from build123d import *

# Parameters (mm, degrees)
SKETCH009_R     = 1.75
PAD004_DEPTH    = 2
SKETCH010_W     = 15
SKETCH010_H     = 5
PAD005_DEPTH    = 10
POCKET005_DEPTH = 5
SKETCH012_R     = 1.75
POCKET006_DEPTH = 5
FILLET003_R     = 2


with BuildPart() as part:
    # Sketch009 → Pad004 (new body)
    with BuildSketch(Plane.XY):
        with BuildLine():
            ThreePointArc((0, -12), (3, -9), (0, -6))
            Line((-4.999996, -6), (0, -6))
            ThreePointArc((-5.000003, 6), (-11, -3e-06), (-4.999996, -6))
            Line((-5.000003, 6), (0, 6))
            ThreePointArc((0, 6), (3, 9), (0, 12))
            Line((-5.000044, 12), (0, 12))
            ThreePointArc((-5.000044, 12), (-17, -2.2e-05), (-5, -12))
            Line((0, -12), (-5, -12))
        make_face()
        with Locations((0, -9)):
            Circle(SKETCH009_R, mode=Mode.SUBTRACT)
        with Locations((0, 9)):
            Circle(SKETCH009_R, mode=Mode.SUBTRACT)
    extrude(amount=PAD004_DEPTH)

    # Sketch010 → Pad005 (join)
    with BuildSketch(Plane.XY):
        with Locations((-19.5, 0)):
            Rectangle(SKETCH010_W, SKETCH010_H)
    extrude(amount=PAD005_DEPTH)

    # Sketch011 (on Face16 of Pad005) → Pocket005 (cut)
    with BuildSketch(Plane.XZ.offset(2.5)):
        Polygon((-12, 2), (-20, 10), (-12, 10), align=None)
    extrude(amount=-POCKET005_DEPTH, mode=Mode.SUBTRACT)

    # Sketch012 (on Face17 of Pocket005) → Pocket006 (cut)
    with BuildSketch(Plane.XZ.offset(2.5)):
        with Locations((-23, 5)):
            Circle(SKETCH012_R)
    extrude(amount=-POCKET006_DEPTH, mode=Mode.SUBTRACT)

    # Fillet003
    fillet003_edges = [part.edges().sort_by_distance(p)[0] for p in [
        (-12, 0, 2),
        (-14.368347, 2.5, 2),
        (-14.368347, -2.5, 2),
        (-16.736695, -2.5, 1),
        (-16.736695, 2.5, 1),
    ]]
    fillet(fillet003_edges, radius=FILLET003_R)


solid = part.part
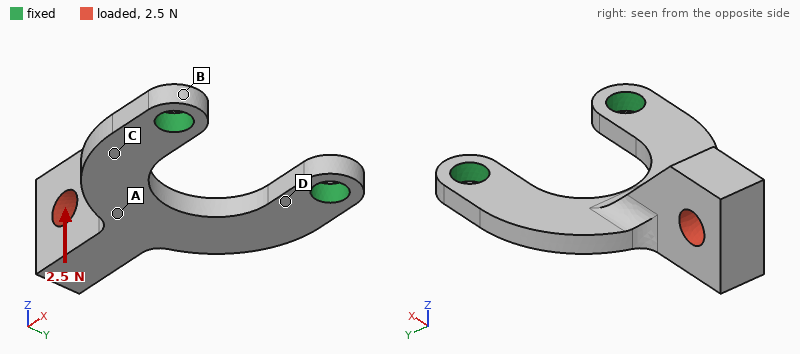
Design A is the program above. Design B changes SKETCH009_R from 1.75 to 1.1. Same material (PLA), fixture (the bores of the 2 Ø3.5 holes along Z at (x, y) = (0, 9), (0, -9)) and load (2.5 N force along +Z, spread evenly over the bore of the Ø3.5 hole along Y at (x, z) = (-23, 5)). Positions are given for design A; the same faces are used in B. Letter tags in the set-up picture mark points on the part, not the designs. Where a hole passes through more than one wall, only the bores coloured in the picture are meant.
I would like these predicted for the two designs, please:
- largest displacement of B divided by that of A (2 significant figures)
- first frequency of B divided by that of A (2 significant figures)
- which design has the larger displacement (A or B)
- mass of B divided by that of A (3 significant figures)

1.1
0.94
B
1.02
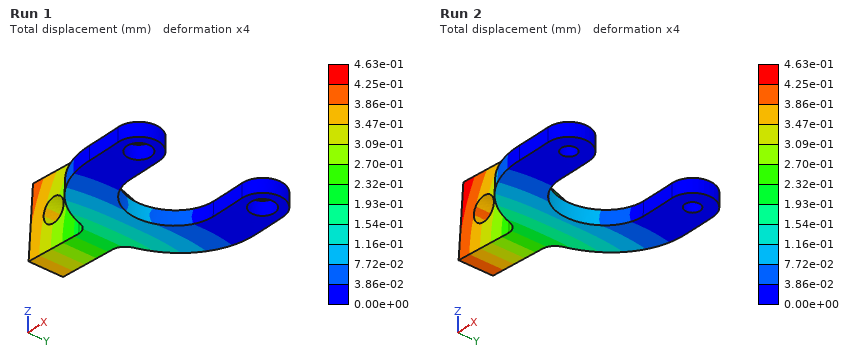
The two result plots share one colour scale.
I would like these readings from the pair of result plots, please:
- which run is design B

Run 2
